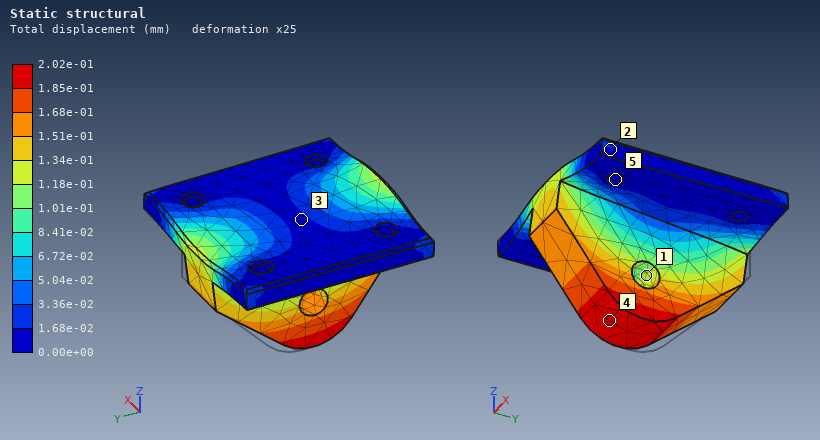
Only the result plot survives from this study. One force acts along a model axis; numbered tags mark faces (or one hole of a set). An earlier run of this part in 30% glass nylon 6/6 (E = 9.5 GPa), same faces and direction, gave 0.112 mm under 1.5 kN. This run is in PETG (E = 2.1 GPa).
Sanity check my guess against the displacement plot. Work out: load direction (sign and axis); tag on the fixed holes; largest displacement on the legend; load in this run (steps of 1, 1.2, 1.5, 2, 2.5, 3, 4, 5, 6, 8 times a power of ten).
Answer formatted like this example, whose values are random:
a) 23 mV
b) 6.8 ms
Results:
a) -Y
b) 5
c) 2.02e-01 mm
d) 600 N
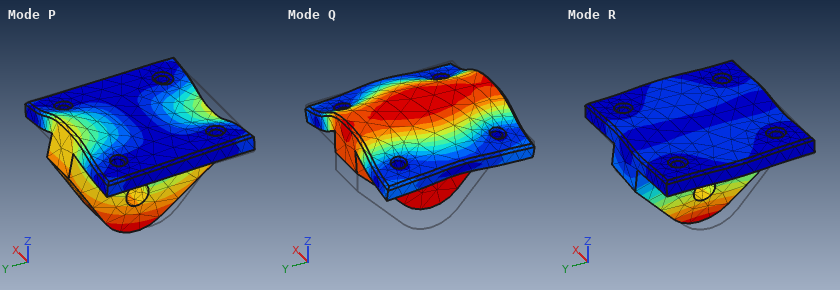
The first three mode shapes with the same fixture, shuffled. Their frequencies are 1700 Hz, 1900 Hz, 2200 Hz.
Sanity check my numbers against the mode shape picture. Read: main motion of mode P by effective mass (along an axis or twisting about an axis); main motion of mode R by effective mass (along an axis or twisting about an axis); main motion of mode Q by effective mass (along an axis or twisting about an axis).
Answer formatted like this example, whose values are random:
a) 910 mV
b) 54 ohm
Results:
a) along Y
b) along X
c) along Z
